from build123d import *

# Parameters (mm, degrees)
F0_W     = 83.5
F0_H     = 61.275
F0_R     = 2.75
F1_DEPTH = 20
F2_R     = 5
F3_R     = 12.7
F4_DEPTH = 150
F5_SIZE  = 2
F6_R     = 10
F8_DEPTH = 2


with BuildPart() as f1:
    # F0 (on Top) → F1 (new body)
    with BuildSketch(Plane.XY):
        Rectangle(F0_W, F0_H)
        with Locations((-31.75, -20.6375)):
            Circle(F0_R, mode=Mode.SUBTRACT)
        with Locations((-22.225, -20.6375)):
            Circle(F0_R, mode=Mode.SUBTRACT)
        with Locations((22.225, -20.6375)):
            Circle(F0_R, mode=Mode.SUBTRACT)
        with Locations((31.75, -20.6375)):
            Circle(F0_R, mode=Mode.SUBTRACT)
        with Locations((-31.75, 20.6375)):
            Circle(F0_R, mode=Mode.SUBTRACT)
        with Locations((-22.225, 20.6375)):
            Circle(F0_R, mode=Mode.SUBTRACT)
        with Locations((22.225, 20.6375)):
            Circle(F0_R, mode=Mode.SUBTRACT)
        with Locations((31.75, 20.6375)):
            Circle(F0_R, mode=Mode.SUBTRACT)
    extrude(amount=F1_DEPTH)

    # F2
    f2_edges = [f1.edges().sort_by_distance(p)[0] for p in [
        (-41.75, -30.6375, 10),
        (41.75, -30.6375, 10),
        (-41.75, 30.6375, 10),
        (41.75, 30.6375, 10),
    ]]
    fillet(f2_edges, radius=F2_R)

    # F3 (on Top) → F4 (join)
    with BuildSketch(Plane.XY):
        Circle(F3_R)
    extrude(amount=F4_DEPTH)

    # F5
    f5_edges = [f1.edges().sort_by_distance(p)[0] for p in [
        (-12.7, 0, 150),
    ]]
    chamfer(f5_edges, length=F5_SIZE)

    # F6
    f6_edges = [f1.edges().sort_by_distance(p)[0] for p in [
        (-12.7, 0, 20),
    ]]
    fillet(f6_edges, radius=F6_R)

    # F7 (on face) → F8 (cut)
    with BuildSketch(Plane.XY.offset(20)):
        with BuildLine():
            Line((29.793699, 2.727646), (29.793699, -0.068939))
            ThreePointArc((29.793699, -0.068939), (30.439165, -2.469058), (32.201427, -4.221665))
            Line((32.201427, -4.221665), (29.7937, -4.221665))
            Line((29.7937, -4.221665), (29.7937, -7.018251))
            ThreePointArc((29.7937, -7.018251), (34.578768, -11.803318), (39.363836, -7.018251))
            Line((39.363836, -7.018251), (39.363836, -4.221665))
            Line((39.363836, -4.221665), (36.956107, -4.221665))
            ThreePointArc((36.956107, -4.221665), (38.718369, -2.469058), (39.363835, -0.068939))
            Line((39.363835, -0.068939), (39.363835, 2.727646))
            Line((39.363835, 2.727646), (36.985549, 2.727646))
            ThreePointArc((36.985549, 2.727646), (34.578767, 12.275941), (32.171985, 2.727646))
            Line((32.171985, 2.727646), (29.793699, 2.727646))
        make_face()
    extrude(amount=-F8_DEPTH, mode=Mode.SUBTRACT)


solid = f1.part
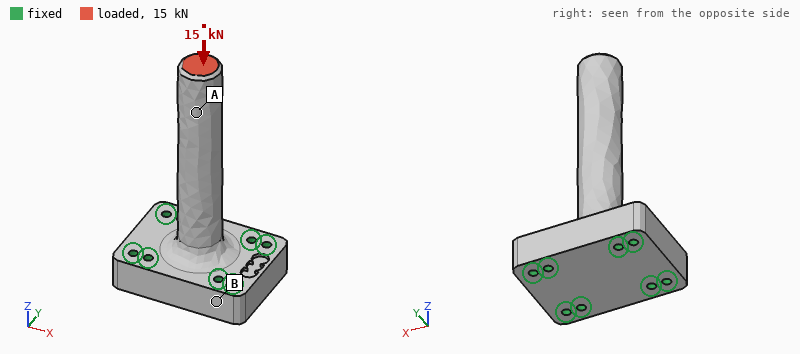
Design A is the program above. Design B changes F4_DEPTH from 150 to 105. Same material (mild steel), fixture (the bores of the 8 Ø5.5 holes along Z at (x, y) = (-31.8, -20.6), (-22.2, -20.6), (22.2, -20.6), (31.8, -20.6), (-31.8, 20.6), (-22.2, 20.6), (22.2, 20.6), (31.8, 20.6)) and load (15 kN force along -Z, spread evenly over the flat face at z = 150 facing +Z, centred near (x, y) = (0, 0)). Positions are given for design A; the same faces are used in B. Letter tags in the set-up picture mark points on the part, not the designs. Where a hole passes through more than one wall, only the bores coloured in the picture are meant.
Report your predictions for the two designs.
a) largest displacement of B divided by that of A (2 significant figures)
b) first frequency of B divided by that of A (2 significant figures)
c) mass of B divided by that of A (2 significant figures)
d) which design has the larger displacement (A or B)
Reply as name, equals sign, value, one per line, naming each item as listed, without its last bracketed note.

largest displacement of B divided by that of A = 0.70
first frequency of B divided by that of A = 2.3
mass of B divided by that of A = 0.86
which design has the larger displacement = A
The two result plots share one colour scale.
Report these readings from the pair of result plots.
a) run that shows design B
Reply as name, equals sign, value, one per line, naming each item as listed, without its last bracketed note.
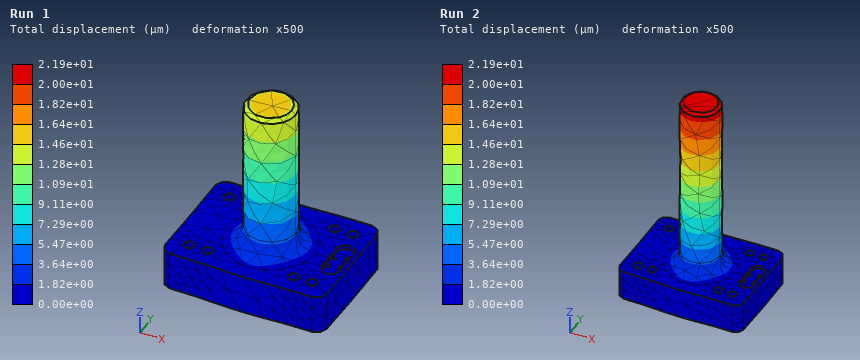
run that shows design B = Run 1
